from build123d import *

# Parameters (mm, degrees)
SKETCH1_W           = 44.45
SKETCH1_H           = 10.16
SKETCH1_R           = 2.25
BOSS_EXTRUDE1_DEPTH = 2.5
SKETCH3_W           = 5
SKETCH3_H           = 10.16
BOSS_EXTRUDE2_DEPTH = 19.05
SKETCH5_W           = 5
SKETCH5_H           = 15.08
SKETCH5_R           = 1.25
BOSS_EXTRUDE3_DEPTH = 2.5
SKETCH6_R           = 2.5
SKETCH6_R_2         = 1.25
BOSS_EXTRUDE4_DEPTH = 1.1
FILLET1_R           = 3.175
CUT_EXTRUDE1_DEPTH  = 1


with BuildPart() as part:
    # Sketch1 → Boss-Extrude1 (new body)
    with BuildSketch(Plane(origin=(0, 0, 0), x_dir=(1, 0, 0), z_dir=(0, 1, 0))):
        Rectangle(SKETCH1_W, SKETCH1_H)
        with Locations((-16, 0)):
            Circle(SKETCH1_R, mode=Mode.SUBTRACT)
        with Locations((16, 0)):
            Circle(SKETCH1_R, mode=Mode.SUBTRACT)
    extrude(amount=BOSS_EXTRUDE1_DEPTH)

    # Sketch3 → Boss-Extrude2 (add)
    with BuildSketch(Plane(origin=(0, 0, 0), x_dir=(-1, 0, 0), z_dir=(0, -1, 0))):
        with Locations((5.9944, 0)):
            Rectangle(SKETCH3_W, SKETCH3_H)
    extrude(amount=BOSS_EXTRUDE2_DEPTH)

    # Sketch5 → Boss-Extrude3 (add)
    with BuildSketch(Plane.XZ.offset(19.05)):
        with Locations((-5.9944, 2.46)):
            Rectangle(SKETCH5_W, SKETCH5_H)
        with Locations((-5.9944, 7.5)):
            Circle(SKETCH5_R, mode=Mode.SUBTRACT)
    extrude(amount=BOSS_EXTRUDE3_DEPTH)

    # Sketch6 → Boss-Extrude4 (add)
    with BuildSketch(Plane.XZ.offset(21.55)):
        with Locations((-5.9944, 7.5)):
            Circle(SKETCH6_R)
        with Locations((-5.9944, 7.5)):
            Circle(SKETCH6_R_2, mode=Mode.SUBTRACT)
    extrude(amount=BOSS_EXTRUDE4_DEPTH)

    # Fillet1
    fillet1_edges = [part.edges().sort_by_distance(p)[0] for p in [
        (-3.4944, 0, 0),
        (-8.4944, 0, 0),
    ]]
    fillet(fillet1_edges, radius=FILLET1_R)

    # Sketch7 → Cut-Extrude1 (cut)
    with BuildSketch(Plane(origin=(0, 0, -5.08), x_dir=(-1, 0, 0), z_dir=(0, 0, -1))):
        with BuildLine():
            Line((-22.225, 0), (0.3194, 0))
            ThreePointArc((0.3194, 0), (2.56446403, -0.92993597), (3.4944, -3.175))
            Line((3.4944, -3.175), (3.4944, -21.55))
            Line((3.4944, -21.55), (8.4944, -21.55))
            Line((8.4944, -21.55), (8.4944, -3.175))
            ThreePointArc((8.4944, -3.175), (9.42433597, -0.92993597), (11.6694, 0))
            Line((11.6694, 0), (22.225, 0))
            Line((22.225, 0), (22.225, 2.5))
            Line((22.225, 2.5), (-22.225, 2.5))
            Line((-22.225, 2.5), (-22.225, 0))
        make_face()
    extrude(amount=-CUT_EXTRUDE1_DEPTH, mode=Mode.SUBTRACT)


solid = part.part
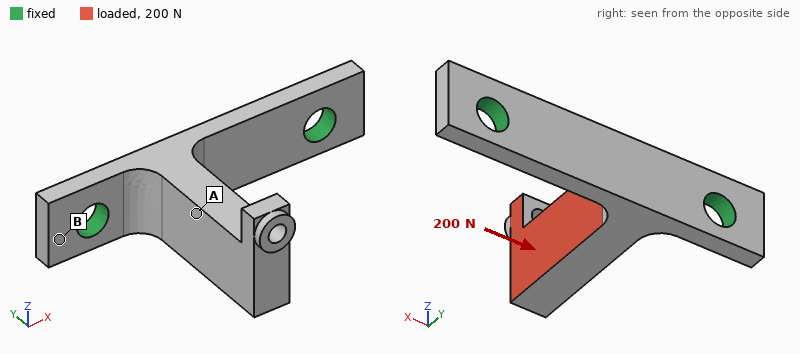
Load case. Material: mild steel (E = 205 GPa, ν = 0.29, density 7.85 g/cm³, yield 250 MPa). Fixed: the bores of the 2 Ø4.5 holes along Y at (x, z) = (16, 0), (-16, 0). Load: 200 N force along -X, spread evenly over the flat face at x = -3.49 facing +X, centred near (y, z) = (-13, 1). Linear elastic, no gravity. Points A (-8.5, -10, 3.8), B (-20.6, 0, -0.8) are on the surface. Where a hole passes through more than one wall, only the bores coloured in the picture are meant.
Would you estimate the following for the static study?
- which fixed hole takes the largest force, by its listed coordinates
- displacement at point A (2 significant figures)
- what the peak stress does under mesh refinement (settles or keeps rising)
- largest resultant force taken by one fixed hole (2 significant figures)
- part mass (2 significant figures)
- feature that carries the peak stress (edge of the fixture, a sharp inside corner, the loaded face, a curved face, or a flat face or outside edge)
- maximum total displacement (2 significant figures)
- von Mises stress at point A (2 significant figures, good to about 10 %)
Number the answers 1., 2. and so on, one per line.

1. (-16, 0)
2. 19 µm
3. keeps rising
4. 170 N
5. 16 g
6. edge of the fixture
7. 48 µm
8. 22 MPa
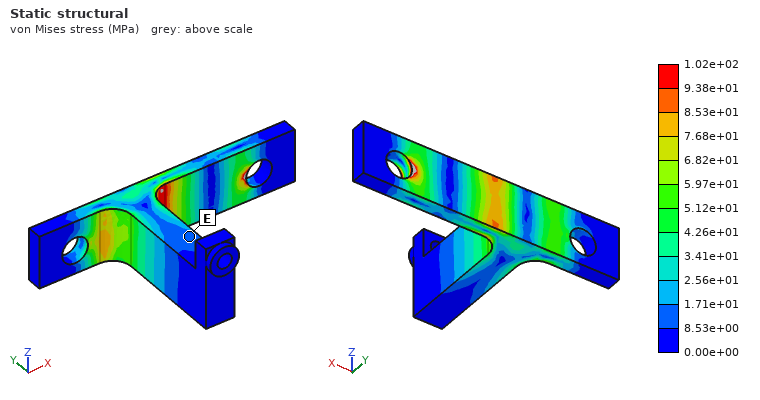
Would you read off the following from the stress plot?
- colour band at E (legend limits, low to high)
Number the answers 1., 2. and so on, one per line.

1. 8.53e+00 to 1.71e+01 MPa
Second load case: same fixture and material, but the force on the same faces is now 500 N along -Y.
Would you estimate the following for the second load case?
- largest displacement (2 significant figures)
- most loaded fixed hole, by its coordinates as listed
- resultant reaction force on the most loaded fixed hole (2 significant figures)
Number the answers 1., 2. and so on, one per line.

1. 58 µm
2. (-16, 0)
3. 340 N
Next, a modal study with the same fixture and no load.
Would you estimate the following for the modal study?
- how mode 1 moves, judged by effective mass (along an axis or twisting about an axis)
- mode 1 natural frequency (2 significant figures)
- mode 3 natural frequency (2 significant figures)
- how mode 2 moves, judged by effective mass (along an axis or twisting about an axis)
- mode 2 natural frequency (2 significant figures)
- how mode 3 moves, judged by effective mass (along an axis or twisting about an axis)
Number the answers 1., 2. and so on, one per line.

1. along Z
2. 3800 Hz
3. 13 kHz
4. along X
5. 4500 Hz
6. along Y
